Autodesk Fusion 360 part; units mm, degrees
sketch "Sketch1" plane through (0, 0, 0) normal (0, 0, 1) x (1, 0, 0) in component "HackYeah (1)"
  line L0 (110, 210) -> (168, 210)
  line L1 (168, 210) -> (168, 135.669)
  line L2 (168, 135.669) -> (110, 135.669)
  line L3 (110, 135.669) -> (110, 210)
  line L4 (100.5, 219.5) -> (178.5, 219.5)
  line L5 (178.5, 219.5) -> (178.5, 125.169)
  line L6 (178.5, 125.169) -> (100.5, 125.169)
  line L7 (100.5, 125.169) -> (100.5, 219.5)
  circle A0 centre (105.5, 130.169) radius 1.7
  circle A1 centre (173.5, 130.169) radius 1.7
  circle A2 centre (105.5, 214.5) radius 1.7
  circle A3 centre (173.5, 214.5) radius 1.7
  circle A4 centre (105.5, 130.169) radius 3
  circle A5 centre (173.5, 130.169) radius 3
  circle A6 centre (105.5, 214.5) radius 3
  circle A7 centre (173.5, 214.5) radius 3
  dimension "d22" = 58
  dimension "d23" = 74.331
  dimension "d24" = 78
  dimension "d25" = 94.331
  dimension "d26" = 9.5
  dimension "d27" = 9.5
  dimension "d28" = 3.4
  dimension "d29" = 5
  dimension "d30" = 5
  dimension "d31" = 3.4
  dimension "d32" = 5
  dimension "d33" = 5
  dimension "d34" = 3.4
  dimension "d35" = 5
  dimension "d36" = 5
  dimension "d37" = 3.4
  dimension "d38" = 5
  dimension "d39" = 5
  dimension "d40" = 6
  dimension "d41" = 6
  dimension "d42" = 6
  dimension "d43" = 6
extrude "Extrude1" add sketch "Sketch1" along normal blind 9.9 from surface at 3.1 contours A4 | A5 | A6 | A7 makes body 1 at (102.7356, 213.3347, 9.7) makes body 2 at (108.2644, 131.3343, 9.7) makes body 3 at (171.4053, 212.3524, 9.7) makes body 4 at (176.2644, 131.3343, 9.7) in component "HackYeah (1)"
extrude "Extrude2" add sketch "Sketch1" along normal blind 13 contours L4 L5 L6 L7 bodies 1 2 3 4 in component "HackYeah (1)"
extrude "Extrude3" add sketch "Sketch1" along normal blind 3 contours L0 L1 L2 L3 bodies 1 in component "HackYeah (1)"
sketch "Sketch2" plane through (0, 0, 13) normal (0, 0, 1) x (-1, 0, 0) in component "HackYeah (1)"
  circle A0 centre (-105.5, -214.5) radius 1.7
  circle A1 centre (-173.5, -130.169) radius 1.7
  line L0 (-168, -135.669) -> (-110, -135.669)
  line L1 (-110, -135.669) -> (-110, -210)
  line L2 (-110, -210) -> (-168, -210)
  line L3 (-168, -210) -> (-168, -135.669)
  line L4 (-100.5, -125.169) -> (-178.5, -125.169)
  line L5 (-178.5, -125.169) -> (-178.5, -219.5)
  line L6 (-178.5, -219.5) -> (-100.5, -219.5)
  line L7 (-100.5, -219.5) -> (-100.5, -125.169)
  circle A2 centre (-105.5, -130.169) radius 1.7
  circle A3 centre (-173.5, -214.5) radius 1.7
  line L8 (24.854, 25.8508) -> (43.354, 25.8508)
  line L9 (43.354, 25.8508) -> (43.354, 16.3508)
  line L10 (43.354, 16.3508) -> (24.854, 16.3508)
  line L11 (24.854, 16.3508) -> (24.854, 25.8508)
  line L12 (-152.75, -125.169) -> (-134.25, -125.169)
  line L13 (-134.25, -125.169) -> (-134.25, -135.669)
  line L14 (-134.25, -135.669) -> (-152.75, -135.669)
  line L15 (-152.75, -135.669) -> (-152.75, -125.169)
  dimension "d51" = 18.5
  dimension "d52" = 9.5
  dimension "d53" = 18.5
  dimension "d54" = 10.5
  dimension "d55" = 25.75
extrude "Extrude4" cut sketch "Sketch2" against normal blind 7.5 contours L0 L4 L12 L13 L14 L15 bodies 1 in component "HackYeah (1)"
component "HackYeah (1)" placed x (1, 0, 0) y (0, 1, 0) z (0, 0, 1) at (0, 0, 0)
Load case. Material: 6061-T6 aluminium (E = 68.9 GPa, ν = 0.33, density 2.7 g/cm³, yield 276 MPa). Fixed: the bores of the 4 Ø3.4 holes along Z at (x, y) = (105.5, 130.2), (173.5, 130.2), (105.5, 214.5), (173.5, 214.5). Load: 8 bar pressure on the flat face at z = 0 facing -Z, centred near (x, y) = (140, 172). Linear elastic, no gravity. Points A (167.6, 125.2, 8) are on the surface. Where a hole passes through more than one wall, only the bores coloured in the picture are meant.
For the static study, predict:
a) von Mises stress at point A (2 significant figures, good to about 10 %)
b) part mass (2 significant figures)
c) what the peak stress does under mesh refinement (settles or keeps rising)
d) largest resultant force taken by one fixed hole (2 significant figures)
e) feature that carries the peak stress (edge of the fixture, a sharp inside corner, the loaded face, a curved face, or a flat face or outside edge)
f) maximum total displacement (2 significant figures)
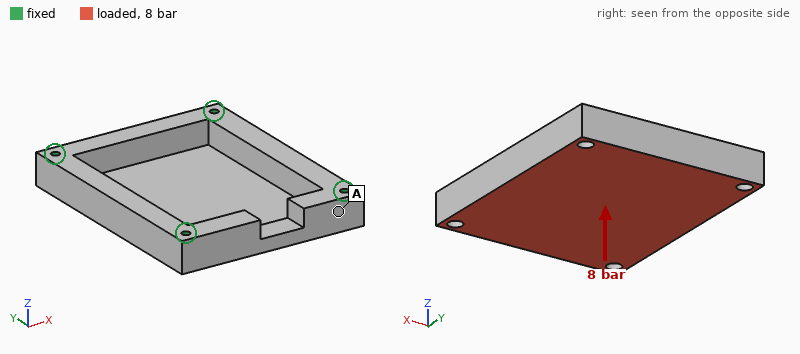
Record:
15 MPa
140 g
keeps rising
2.2 kN
edge of the fixture
0.19 mm
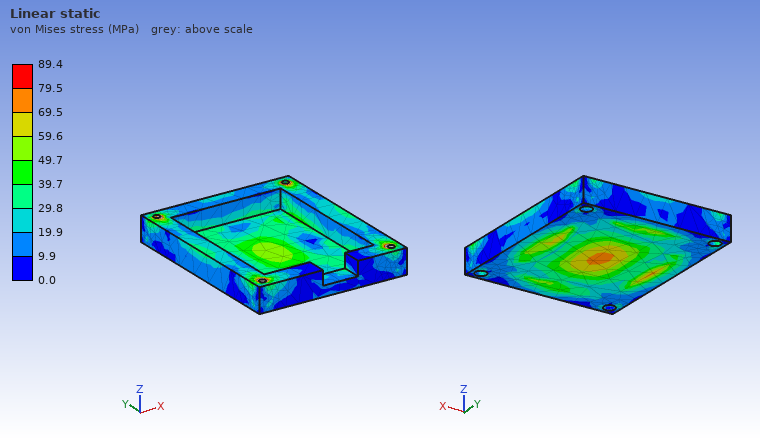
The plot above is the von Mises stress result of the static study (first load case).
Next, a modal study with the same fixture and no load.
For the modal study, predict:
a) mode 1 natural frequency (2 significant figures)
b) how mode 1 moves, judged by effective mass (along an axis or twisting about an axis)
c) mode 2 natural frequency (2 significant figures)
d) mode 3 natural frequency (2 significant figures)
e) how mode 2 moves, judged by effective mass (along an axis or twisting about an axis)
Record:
4600 Hz
along Z
6900 Hz
8100 Hz
twisting about Y
